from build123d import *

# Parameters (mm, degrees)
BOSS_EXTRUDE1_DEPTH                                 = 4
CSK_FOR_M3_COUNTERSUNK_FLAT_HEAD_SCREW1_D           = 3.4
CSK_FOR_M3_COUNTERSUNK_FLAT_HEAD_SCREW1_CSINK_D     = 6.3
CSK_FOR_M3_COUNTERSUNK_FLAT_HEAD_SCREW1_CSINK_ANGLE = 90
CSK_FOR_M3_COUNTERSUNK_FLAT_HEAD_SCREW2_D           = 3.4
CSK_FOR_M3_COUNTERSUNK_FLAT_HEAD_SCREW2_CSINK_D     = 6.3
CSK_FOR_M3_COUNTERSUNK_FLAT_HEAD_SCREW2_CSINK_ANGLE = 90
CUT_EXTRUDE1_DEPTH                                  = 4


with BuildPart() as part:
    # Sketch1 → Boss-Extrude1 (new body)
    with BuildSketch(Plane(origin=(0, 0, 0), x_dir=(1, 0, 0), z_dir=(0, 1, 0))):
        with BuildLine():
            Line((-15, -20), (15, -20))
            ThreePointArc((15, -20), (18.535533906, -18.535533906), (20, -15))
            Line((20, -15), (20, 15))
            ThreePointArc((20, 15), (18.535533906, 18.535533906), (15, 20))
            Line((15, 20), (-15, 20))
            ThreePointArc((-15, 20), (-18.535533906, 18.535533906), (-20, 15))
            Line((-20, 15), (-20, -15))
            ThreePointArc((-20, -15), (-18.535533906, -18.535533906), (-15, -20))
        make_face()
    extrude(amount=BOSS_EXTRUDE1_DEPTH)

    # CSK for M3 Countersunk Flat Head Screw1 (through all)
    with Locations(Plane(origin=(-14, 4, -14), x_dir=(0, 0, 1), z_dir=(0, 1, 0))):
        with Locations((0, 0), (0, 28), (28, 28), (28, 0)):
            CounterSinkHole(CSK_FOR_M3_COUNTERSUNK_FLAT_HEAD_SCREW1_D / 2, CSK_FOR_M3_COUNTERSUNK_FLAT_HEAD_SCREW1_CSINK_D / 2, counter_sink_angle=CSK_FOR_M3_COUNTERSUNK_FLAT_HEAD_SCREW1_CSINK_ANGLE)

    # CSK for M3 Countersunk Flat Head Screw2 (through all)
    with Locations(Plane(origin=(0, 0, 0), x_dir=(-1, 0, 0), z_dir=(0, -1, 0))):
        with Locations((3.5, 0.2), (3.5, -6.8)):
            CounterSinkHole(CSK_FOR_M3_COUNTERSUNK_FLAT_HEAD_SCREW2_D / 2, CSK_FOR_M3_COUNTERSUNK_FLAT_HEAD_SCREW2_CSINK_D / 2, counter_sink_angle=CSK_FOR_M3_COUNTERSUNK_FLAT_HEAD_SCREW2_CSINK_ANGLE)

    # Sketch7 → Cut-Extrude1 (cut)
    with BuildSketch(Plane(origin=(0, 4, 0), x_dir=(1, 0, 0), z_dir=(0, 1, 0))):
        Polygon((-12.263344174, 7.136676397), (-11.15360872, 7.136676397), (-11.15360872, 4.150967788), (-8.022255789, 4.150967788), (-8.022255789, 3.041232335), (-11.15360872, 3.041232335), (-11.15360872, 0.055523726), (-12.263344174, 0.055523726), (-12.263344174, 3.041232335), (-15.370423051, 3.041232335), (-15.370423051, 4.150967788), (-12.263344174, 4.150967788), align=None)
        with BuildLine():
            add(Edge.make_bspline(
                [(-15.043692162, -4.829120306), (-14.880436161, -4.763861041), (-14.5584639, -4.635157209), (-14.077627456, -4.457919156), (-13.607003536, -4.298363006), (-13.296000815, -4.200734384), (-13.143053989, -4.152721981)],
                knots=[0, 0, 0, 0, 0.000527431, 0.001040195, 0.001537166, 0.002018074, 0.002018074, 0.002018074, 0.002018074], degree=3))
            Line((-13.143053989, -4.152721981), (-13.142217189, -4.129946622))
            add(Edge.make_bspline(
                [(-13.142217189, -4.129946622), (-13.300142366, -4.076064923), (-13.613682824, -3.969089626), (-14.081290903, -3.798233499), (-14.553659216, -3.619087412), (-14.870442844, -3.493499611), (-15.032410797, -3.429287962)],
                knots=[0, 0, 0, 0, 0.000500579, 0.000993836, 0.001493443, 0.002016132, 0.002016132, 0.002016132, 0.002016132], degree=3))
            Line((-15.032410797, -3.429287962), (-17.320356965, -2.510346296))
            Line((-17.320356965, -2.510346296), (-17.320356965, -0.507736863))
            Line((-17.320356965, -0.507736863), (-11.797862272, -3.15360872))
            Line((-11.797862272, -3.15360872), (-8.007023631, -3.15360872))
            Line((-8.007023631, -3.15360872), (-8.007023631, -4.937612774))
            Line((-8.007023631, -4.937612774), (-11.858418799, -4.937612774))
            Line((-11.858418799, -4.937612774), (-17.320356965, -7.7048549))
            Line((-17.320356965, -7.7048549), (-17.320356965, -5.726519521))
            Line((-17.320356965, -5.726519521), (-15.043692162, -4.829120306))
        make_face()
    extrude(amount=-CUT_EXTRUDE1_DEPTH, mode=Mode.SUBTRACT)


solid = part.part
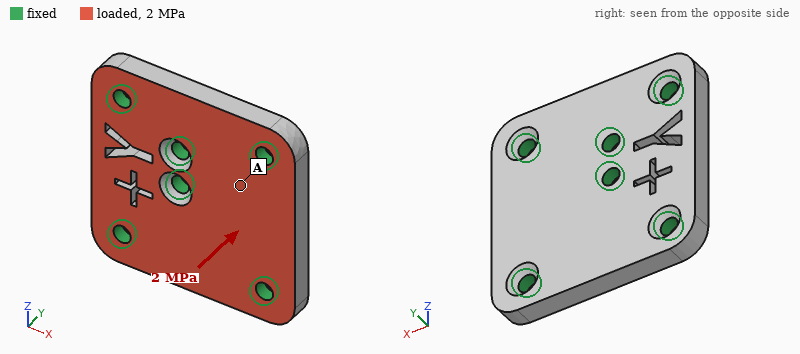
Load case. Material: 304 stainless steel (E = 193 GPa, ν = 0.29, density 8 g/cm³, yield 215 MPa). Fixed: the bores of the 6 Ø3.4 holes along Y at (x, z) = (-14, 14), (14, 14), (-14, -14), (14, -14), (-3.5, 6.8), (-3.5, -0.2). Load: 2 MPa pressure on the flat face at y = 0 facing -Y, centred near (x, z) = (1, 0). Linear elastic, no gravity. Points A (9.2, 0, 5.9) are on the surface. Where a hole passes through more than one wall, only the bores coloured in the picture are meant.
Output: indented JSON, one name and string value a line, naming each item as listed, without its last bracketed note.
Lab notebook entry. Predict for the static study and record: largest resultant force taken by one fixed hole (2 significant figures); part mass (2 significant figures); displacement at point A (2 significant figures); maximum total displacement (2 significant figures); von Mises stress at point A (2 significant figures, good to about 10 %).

{
  "largest resultant force taken by one fixed hole": "630 N",
  "part mass": "47 g",
  "displacement at point A": "2.4 µm",
  "maximum total displacement": "4.6 µm",
  "von Mises stress at point A": "14 MPa"
}
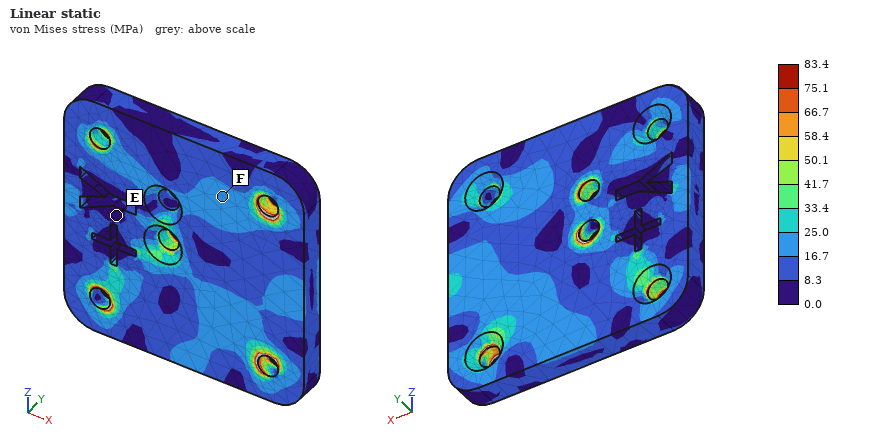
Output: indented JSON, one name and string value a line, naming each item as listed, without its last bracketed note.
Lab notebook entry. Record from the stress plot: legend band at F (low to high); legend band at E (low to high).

{
  "legend band at F": "16.7 to 25.0 MPa",
  "legend band at E": "0.0 to 8.3 MPa"
}
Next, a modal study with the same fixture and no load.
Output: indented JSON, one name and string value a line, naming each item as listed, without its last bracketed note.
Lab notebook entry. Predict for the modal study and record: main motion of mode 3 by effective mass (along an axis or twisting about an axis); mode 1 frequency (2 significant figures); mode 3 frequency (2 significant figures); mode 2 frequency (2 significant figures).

{
  "main motion of mode 3 by effective mass": "along Y",
  "mode 1 frequency": "22 kHz",
  "mode 3 frequency": "24 kHz",
  "mode 2 frequency": "22 kHz"
}
